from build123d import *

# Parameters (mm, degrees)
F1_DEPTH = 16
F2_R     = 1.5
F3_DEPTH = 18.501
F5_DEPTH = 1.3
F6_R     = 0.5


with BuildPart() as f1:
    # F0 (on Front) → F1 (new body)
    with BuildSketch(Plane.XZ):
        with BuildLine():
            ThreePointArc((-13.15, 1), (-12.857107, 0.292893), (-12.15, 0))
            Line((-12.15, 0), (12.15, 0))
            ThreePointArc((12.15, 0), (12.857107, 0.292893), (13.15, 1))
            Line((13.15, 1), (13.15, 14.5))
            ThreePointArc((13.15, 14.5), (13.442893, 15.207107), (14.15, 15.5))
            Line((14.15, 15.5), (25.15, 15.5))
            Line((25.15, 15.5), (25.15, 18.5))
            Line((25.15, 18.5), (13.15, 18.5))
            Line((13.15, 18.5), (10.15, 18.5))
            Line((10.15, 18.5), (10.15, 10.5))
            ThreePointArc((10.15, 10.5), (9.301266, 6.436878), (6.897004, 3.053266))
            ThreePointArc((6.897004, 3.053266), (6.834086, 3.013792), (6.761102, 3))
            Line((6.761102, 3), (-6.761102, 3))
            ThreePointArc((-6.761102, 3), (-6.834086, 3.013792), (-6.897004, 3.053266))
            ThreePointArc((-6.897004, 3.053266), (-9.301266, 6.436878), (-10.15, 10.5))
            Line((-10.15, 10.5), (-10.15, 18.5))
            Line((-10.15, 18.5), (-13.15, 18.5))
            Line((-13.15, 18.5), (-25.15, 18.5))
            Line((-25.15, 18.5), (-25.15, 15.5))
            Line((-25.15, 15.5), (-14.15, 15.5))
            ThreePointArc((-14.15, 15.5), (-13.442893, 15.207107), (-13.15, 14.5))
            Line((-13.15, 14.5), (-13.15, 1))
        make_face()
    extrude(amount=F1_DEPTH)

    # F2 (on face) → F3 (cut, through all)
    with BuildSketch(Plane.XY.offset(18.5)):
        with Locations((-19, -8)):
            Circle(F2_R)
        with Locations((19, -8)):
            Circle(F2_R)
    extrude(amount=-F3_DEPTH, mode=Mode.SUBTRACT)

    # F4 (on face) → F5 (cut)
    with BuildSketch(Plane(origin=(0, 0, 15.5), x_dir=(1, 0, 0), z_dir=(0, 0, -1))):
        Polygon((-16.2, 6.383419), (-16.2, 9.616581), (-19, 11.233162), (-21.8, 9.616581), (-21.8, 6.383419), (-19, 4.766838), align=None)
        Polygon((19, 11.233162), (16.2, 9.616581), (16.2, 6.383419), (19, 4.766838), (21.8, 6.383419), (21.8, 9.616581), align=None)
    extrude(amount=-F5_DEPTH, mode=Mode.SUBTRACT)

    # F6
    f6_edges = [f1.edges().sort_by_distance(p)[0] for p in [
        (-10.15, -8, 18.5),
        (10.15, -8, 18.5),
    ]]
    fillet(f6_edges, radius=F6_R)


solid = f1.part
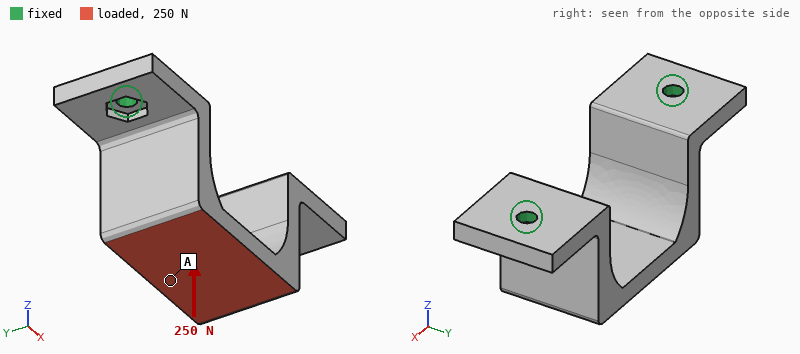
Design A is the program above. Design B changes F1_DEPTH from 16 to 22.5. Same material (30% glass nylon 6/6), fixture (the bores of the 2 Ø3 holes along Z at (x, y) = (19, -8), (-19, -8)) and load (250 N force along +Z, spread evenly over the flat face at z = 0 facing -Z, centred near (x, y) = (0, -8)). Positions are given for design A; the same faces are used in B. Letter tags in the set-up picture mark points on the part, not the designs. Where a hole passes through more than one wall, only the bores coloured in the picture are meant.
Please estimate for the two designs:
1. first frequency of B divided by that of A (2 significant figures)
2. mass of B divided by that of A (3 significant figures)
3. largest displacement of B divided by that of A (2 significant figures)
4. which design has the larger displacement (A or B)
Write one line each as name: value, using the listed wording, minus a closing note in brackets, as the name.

first frequency of B divided by that of A: 0.80
mass of B divided by that of A: 1.42
largest displacement of B divided by that of A: 4.2
which design has the larger displacement: B
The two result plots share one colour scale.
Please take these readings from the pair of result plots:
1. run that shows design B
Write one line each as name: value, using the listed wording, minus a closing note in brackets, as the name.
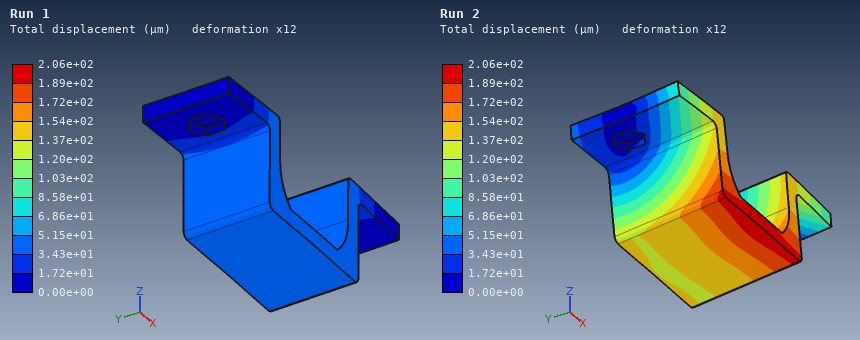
run that shows design B: Run 2
